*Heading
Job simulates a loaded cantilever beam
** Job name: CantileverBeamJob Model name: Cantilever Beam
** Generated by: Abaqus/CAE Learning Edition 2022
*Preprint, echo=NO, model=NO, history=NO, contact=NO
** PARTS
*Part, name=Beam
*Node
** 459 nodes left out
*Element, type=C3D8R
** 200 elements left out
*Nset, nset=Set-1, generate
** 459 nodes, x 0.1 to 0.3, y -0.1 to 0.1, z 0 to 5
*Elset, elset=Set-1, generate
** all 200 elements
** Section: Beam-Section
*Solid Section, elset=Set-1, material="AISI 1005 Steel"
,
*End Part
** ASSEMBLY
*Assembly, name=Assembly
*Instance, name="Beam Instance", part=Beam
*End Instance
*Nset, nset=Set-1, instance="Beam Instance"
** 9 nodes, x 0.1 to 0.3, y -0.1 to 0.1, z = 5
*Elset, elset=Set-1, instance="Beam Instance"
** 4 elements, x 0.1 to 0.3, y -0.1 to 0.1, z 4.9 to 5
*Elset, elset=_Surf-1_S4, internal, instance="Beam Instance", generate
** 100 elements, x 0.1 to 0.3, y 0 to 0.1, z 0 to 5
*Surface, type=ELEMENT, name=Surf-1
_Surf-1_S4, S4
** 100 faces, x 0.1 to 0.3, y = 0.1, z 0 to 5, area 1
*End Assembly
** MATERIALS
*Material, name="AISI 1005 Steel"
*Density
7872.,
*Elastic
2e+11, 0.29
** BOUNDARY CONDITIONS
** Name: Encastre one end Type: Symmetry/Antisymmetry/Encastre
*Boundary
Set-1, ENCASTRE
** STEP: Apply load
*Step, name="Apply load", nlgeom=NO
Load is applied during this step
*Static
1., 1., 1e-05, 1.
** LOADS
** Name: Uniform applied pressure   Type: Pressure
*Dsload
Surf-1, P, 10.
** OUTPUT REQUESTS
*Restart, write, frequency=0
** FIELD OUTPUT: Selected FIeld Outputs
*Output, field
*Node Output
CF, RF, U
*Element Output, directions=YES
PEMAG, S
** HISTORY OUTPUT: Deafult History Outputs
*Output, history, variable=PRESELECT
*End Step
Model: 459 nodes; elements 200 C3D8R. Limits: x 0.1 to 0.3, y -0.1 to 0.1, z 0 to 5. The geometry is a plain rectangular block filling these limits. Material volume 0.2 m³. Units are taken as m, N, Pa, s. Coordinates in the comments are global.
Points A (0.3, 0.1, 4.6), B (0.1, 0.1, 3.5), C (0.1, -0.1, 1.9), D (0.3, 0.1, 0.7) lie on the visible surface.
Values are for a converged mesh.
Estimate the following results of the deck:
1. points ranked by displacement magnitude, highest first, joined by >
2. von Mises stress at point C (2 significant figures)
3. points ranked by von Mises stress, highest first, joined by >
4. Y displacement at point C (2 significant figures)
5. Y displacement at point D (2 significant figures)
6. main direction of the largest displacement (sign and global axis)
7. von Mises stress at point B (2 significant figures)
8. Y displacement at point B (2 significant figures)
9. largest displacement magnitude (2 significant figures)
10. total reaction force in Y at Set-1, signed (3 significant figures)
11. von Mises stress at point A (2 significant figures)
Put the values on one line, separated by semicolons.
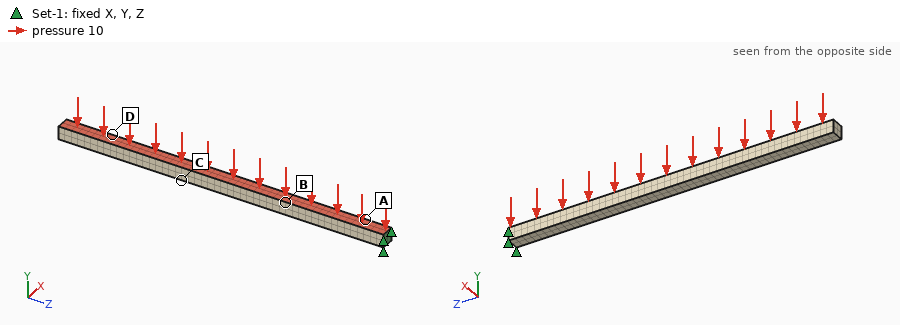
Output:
D > C > B > A; 2700 Pa; A > B > C > D; -2.9e-06 m; -4.8e-06 m; -Y; 9200 Pa; -8.6e-07 m; 5.8e-06 m; 10.0 N; 16000 Pa
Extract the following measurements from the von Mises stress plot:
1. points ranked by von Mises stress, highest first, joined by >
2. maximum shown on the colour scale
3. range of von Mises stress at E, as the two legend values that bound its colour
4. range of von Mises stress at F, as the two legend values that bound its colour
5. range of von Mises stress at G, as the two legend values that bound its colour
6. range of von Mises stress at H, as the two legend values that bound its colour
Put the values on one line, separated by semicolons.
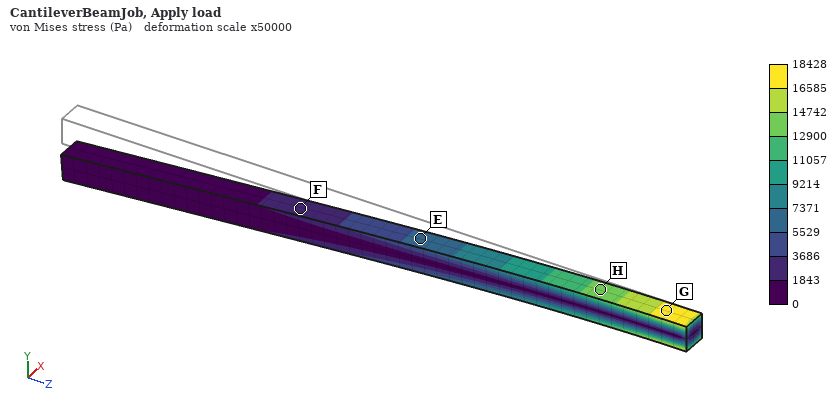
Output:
G > H > E > F; 18428 Pa; 5529 to 7371 Pa; 1843 to 3686 Pa; 16585 to 18428 Pa; 12900 to 14742 Pa
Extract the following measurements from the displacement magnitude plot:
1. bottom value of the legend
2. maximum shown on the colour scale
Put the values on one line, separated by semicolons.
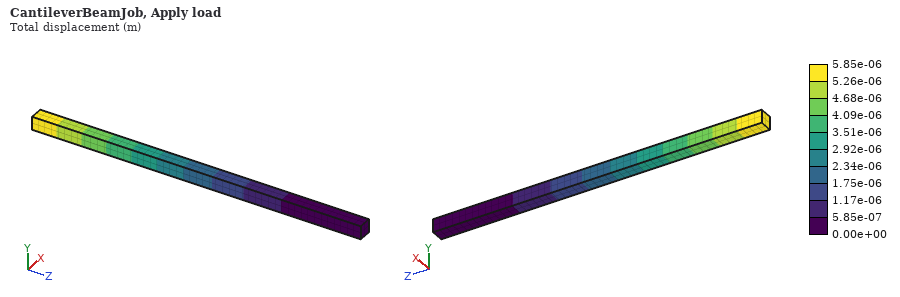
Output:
0.00e+00 m; 5.85e-06 m
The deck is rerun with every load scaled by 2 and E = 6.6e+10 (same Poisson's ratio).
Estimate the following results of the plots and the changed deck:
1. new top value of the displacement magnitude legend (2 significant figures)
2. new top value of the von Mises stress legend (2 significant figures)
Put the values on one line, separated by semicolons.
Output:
3.5e-05 m; 37000 Pa
